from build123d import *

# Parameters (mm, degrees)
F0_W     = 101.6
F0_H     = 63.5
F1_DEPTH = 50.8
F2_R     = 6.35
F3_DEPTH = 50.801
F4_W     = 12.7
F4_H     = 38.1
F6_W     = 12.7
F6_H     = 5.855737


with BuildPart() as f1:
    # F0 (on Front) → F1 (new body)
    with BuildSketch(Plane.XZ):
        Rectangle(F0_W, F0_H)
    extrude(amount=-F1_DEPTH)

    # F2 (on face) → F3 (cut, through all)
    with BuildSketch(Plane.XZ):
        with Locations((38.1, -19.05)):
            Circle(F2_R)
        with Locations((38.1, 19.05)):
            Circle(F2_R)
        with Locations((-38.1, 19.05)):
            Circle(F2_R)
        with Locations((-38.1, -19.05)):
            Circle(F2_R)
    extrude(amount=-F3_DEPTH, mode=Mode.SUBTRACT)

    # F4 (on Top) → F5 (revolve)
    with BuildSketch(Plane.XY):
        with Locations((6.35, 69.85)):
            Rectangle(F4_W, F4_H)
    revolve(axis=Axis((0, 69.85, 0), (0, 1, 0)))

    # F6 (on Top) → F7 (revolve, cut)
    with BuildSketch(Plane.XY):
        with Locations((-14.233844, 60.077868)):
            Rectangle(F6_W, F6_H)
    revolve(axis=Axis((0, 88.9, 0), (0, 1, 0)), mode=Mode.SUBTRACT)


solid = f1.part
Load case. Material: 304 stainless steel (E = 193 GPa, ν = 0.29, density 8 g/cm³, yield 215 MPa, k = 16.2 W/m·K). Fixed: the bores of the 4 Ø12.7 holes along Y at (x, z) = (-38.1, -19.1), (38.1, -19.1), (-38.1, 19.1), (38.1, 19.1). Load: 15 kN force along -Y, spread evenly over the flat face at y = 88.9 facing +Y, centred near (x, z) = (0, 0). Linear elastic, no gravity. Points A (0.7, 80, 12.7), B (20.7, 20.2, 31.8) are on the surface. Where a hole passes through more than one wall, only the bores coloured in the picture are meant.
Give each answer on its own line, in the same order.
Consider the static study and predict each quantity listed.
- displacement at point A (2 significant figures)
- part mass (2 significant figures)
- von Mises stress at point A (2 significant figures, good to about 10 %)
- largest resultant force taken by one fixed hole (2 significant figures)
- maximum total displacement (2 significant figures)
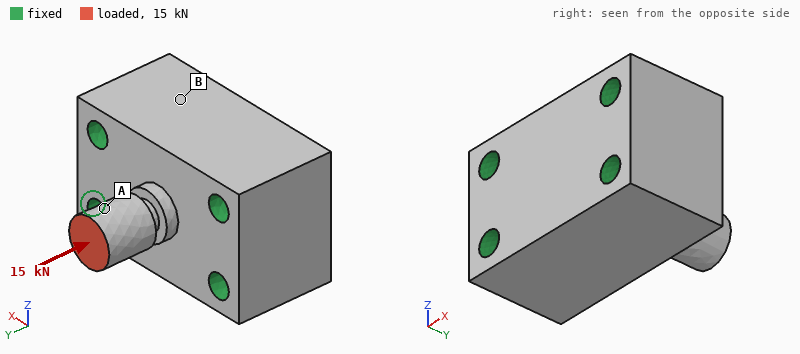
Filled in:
10 µm
2.6 kg
29 MPa
3.9 kN
12 µm
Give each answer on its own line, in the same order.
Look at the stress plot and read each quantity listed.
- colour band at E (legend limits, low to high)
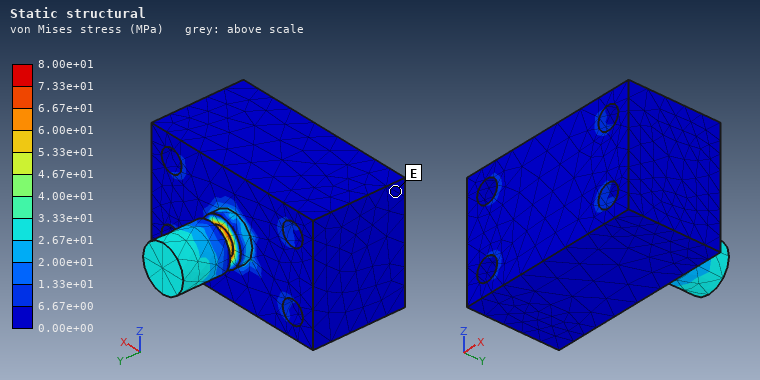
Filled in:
0.00e+00 to 6.67e+00 MPa
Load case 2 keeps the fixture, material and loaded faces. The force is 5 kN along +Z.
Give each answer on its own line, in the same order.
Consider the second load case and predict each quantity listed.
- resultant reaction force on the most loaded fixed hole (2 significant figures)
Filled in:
3.1 kN
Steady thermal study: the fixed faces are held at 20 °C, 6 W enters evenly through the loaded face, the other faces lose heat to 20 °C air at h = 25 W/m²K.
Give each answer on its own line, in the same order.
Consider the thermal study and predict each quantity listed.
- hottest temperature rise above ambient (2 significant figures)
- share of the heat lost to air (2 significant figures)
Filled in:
37 K
34 %
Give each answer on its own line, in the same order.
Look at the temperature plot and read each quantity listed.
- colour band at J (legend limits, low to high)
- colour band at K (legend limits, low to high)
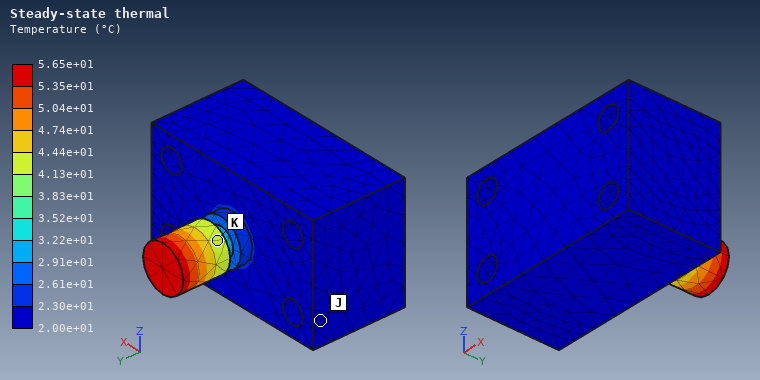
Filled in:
2.00e+01 to 2.30e+01 °C
4.13e+01 to 4.44e+01 °C
